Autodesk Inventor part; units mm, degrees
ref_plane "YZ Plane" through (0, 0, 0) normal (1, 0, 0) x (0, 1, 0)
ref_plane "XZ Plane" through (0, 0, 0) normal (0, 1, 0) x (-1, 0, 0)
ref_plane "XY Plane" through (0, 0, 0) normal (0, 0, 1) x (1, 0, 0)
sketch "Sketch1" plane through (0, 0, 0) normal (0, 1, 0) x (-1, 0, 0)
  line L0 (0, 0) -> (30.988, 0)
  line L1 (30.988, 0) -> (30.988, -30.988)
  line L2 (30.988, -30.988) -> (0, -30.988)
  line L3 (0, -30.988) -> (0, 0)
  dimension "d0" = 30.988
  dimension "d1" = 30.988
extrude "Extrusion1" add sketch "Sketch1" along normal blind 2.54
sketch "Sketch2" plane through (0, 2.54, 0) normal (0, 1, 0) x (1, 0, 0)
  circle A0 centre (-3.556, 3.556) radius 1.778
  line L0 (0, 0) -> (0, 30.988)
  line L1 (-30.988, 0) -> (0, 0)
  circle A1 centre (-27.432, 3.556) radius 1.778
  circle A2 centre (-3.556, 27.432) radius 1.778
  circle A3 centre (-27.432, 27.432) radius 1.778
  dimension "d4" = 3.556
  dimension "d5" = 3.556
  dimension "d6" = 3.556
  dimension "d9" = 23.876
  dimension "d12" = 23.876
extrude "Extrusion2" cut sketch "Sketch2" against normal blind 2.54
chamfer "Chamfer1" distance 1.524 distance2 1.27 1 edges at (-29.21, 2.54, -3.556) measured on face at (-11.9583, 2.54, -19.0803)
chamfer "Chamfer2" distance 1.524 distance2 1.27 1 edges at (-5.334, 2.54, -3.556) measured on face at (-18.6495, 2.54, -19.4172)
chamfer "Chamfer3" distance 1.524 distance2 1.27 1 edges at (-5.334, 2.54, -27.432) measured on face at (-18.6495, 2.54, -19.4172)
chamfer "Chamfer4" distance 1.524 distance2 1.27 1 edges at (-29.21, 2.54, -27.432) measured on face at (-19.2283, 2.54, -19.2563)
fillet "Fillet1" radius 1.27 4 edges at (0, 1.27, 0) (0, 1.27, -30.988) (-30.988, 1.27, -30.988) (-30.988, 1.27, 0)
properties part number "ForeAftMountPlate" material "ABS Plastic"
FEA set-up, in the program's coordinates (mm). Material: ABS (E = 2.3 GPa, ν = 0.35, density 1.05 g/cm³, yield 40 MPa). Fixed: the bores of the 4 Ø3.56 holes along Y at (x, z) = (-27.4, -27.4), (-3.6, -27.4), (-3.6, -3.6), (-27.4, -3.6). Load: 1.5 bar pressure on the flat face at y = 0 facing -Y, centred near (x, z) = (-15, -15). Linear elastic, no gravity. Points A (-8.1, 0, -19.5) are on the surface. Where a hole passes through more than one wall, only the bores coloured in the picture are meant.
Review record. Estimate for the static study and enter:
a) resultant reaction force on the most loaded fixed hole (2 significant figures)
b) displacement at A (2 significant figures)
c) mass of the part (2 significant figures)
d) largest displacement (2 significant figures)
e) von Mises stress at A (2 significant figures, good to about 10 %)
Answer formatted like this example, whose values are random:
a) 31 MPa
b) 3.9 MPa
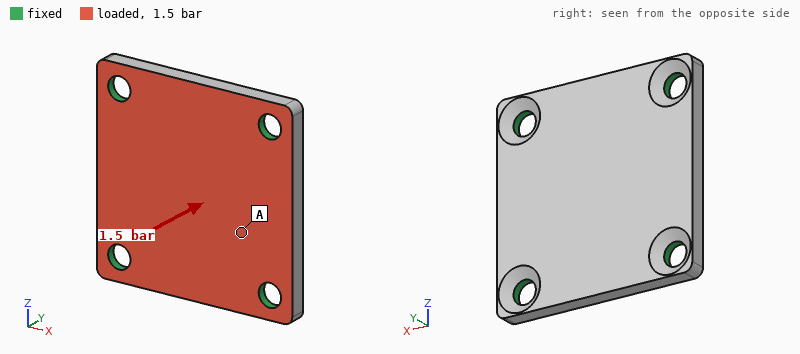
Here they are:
a) 42 N
b) 0.074 mm
c) 2.4 g
d) 0.11 mm
e) 2.4 MPa
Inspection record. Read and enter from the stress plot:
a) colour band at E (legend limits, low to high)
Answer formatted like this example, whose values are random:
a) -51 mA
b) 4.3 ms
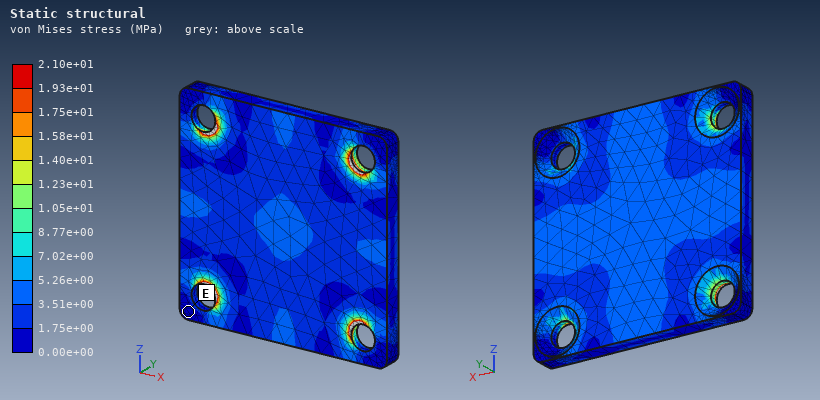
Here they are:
a) 0.00e+00 to 1.75e+00 MPa
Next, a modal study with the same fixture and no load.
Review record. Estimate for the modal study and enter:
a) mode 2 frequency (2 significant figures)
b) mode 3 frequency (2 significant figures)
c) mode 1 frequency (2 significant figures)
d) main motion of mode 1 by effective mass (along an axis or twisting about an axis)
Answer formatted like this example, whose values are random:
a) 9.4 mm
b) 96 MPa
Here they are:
a) 6800 Hz
b) 6800 Hz
c) 4400 Hz
d) along Y
